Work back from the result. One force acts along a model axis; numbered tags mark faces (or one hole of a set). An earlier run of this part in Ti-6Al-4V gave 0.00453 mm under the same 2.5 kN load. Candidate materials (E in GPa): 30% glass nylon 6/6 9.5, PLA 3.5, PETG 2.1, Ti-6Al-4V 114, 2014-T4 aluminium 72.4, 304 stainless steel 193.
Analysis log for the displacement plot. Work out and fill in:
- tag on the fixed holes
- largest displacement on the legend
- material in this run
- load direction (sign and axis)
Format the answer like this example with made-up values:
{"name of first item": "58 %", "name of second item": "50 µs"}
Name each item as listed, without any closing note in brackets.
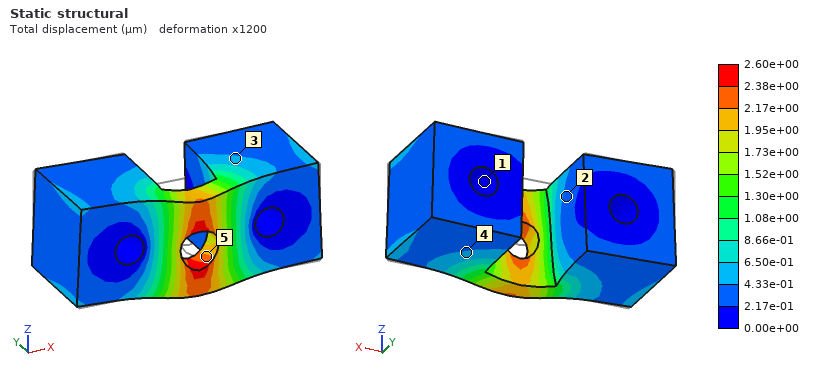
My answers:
{"tag on the fixed holes": "1", "largest displacement on the legend": "2.60e+00 µm", "material in this run": "304 stainless steel", "load direction": "-Z"}
